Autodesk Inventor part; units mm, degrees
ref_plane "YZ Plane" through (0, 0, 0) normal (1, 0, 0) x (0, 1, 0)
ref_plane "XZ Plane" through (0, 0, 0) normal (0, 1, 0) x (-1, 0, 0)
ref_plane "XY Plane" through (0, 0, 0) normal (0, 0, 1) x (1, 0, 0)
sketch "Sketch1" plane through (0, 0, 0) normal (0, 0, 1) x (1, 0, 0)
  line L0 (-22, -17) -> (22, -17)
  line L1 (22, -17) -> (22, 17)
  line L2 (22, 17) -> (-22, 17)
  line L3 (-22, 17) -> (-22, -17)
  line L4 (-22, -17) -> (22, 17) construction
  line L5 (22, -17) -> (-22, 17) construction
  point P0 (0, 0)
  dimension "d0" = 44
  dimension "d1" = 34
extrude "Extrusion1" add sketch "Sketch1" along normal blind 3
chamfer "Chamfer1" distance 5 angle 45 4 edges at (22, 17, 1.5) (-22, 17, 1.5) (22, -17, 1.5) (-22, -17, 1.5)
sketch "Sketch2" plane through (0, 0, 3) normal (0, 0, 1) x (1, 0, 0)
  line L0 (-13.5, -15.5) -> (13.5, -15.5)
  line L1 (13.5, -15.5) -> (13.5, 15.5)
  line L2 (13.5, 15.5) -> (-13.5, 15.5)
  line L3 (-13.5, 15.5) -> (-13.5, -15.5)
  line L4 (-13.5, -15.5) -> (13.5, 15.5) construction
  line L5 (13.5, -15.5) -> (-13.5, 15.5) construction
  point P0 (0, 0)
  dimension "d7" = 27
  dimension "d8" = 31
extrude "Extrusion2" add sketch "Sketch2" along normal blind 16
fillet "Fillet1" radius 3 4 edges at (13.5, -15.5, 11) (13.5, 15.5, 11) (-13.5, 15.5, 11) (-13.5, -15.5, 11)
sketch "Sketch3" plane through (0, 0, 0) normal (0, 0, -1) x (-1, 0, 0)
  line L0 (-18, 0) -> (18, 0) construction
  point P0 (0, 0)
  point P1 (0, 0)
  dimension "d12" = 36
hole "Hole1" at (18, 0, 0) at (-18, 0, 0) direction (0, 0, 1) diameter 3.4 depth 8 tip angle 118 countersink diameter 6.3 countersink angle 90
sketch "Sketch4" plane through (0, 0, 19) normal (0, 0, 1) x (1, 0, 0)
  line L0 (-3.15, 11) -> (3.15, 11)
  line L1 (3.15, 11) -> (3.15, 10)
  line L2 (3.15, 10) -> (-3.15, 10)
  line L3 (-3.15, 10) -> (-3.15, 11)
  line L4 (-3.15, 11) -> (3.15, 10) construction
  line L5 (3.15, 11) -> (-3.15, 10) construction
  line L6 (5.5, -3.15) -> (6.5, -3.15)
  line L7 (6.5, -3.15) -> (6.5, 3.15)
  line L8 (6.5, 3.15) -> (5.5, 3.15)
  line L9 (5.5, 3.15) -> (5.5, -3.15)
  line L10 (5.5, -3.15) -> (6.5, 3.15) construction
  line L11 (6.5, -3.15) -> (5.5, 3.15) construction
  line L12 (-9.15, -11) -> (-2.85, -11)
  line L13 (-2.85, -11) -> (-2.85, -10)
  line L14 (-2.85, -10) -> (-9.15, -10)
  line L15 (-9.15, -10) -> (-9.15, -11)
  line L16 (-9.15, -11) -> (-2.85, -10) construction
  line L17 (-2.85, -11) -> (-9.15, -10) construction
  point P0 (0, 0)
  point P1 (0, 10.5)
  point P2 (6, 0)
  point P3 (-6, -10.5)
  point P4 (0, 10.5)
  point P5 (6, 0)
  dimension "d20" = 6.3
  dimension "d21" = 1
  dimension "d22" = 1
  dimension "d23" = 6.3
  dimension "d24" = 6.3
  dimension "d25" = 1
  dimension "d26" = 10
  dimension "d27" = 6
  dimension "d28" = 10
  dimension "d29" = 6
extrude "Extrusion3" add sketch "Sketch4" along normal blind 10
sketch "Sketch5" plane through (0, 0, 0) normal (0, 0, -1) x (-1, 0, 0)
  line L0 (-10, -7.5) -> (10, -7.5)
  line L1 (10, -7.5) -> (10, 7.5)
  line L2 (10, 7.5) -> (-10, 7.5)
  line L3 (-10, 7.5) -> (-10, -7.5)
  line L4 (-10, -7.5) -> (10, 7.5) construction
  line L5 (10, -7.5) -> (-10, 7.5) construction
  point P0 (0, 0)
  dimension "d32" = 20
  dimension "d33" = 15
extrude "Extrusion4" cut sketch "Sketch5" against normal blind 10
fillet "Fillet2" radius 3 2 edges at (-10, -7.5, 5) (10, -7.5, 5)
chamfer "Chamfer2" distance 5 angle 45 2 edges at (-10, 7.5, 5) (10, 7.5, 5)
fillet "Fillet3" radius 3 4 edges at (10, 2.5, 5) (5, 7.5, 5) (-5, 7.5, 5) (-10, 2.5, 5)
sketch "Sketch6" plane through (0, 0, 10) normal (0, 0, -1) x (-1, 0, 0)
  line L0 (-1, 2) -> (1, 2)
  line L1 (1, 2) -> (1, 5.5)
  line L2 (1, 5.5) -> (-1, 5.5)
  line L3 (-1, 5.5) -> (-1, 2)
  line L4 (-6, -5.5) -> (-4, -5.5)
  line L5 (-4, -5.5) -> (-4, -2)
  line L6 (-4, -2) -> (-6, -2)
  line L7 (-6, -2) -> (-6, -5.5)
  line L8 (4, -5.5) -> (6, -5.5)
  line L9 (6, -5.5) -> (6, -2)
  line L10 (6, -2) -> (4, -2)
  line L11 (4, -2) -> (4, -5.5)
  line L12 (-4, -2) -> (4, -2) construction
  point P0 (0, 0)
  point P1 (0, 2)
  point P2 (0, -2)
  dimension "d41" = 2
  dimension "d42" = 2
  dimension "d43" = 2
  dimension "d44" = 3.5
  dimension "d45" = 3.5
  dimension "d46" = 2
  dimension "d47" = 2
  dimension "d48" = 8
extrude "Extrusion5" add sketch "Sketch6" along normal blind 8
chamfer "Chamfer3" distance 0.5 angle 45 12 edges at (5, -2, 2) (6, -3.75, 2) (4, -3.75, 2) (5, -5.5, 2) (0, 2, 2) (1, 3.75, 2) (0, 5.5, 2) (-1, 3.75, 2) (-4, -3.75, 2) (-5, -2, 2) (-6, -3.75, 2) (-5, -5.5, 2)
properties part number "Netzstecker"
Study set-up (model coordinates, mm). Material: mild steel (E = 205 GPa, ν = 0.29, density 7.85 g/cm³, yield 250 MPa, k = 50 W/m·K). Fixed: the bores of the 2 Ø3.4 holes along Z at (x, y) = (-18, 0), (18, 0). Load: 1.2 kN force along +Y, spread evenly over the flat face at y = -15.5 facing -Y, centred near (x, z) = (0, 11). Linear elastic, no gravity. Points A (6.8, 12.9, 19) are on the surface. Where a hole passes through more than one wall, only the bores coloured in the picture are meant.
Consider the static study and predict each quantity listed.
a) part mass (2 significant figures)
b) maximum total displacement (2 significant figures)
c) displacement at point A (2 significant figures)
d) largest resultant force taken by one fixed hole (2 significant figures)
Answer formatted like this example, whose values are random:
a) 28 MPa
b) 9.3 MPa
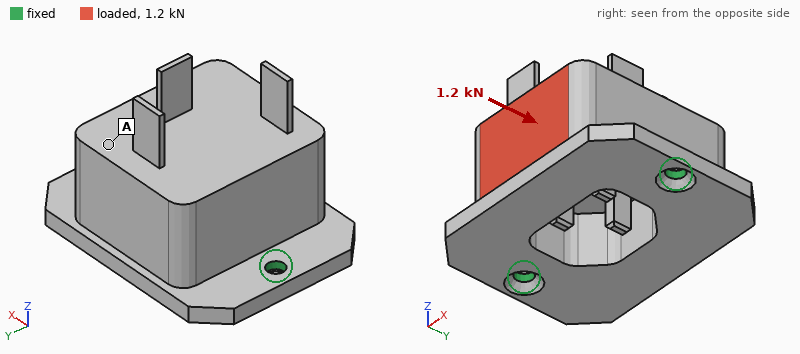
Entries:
a) 120 g
b) 98 µm
c) 72 µm
d) 600 N
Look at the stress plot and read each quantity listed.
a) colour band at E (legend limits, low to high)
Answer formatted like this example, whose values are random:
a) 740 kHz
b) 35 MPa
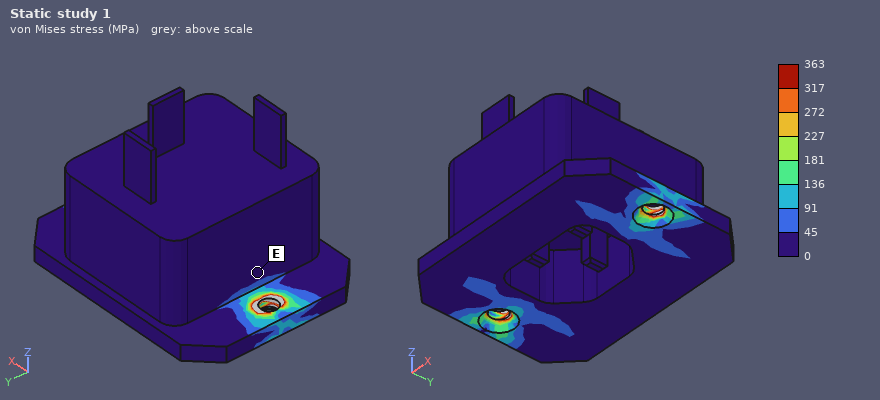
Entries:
a) 0 to 45 MPa
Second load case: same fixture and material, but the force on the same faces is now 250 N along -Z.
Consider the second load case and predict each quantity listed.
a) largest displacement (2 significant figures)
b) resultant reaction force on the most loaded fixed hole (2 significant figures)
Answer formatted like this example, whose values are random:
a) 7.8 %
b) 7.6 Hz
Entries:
a) 35 µm
b) 140 N
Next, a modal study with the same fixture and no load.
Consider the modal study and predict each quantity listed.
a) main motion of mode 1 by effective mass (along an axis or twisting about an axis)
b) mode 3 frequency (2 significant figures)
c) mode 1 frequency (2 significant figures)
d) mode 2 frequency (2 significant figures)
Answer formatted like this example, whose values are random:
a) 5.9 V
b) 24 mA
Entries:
a) along Y
b) 7900 Hz
c) 1900 Hz
d) 7600 Hz
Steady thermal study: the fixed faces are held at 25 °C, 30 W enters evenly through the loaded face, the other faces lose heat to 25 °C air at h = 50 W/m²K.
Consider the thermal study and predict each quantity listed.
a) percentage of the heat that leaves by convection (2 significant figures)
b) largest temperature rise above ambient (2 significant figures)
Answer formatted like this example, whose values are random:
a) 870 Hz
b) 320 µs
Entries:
a) 34 %
b) 59 K
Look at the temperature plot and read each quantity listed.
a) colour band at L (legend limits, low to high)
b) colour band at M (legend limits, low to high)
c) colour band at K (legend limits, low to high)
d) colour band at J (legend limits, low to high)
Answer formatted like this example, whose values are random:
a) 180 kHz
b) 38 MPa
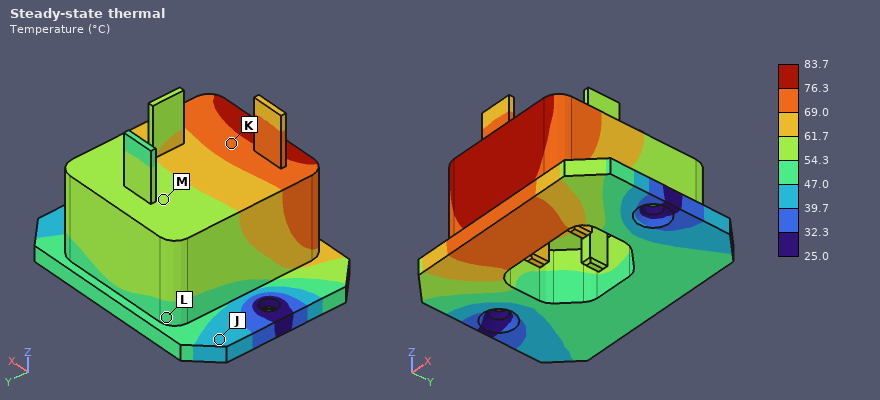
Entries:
a) 47.0 to 54.3 °C
b) 54.3 to 61.7 °C
c) 69.0 to 76.3 °C
d) 39.7 to 47.0 °C
